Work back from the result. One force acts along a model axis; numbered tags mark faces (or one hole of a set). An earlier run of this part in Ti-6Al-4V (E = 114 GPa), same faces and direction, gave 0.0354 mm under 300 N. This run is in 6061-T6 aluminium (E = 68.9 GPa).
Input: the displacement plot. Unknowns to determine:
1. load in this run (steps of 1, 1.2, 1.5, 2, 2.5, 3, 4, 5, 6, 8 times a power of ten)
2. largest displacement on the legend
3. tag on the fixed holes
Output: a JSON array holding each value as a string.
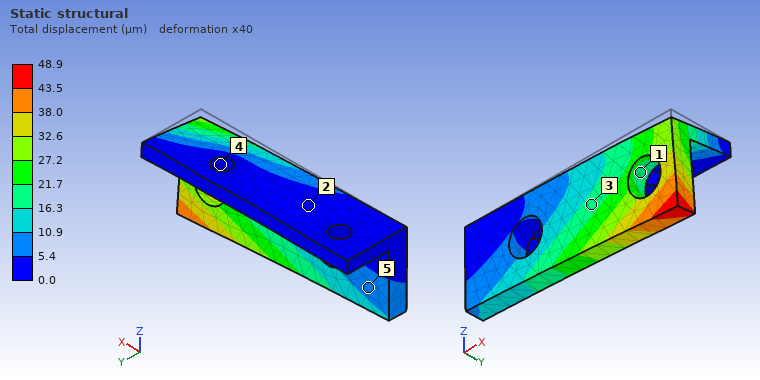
["250 N", "48.9 µm", "4"]
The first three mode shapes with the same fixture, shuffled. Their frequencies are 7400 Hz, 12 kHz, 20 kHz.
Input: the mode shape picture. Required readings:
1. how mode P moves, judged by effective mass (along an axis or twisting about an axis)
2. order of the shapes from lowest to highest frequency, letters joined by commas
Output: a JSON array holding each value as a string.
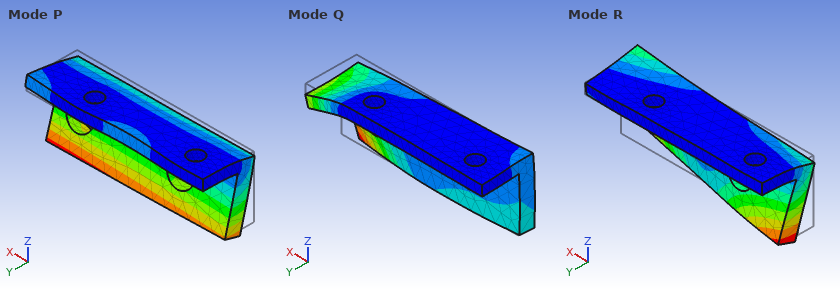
["along Y", "P, R, Q"]
